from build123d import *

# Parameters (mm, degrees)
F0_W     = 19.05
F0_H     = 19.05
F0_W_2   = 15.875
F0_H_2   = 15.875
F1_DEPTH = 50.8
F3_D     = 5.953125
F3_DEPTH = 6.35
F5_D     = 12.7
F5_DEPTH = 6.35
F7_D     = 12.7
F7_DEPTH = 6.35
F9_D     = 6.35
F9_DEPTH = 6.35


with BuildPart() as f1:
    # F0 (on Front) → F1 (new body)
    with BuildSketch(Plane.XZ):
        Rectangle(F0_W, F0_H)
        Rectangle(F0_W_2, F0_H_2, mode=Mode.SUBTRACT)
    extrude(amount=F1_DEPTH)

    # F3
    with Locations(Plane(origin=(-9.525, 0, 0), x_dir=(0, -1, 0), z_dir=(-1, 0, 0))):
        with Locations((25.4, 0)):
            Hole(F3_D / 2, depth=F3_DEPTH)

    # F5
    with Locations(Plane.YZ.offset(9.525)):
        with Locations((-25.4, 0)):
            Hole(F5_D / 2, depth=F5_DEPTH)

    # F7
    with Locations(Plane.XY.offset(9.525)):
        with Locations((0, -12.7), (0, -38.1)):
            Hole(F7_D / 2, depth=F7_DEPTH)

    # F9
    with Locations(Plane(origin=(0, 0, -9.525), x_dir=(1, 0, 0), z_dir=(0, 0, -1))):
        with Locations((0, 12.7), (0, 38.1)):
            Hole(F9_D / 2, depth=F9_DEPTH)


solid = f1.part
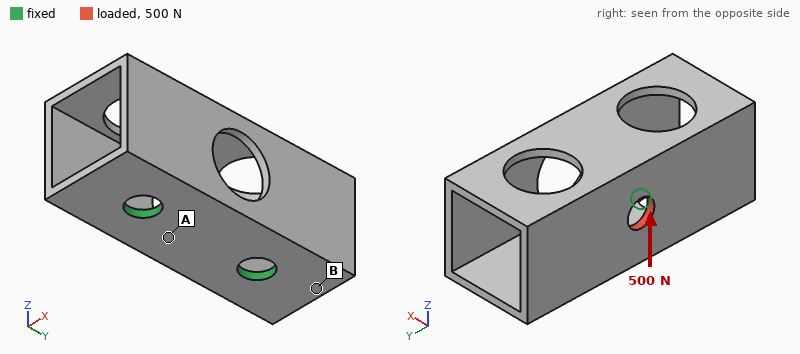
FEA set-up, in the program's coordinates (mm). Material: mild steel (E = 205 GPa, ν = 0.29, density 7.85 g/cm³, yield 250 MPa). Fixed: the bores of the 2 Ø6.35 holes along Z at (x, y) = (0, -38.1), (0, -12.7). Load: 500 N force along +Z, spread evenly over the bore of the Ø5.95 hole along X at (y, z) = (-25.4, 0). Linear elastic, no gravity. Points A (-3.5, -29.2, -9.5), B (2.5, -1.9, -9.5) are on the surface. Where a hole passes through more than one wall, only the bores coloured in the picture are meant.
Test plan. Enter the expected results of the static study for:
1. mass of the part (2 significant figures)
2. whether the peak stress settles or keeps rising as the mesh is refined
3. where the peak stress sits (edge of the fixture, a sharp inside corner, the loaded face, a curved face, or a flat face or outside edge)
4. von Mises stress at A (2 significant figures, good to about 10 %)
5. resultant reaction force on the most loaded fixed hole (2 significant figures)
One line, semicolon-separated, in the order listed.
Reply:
38 g; keeps rising; edge of the fixture; 41 MPa; 260 N
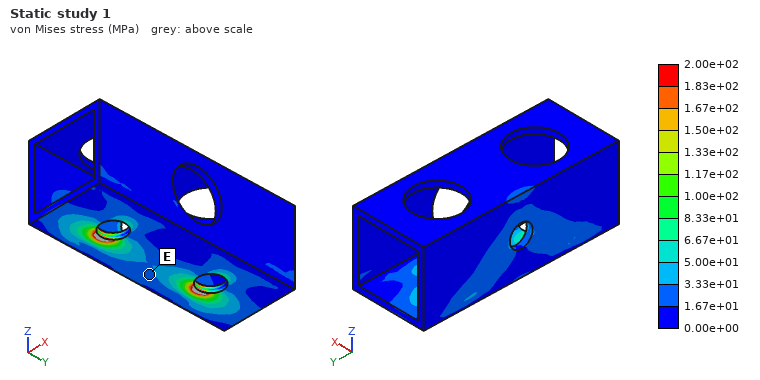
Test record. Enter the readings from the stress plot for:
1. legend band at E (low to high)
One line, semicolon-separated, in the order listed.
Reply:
1.67e+01 to 3.33e+01 MPa
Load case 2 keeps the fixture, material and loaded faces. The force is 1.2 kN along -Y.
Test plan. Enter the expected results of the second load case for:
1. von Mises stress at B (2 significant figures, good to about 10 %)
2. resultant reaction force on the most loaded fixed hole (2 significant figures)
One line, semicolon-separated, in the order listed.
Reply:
48 MPa; 760 N
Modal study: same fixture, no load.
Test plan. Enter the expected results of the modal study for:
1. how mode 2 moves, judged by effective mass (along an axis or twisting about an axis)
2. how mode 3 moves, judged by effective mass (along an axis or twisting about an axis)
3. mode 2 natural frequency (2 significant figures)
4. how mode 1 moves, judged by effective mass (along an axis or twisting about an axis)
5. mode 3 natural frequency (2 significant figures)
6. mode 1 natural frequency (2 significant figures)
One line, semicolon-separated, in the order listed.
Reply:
along Y; twisting about Z; 5700 Hz; along X; 6800 Hz; 2400 Hz
